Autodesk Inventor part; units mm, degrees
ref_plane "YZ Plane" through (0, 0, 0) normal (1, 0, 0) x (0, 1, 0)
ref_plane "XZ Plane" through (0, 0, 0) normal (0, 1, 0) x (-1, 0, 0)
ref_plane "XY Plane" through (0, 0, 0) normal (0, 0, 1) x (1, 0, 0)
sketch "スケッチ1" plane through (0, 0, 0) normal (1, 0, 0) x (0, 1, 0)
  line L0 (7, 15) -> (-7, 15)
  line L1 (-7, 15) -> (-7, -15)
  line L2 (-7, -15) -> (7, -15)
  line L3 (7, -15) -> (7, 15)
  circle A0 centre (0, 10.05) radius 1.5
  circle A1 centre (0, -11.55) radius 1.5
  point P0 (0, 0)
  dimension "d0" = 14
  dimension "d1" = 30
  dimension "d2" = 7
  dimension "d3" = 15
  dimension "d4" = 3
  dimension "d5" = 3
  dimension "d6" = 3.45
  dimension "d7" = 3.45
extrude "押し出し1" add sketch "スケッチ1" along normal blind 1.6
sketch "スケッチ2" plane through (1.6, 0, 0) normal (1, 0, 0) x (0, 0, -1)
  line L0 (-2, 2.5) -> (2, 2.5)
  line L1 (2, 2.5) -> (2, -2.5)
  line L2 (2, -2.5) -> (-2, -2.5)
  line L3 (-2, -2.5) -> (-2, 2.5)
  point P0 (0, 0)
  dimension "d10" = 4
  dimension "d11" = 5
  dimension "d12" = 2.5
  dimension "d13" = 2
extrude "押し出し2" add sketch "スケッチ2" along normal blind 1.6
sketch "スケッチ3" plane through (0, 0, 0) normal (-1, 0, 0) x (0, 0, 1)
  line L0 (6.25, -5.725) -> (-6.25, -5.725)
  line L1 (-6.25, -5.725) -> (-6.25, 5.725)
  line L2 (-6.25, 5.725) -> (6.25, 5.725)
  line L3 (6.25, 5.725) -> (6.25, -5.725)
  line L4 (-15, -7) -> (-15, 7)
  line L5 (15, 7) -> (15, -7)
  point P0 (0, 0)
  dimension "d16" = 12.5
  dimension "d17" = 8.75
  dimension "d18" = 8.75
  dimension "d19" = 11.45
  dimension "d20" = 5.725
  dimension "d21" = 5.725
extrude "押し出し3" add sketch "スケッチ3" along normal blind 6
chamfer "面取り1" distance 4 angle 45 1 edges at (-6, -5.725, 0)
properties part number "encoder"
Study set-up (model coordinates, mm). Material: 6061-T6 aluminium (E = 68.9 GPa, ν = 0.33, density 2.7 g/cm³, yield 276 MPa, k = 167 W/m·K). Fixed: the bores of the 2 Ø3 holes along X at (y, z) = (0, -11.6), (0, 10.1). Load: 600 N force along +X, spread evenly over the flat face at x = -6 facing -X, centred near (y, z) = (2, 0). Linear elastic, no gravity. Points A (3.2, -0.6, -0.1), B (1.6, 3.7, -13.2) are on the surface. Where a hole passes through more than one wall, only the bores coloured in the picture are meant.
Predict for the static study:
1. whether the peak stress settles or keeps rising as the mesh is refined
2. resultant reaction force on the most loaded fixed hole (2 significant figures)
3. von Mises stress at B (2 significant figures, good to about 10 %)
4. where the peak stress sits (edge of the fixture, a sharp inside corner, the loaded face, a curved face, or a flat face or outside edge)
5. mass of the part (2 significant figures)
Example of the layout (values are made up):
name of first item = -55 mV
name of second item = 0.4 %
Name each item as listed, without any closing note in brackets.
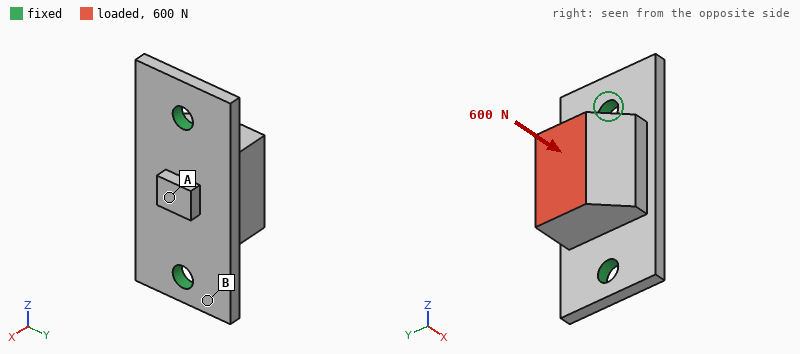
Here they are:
whether the peak stress settles or keeps rising as the mesh is refined = keeps rising
resultant reaction force on the most loaded fixed hole = 350 N
von Mises stress at B = 59 MPa
where the peak stress sits = edge of the fixture
mass of the part = 3.9 g
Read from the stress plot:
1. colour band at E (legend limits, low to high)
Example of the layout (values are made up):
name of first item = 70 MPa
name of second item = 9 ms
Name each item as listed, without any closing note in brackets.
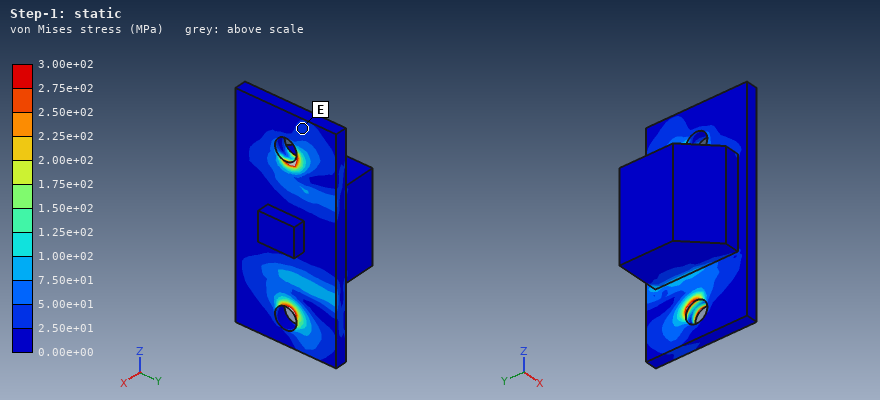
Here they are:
colour band at E = 2.50e+01 to 5.00e+01 MPa
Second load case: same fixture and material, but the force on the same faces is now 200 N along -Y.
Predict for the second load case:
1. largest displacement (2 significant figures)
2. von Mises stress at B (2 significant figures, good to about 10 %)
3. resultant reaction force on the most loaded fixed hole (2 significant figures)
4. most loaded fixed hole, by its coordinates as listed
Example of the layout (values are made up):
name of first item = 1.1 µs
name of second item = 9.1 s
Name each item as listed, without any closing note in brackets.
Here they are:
largest displacement = 38 µm
von Mises stress at B = 37 MPa
resultant reaction force on the most loaded fixed hole = 110 N
most loaded fixed hole, by its coordinates as listed = (0, 10.1)
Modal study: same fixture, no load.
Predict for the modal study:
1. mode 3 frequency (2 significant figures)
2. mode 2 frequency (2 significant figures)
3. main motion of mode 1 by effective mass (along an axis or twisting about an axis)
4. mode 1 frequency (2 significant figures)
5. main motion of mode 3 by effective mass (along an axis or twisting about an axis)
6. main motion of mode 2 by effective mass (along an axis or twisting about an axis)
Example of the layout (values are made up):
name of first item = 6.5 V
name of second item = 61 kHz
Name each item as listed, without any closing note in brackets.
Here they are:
mode 3 frequency = 30 kHz
mode 2 frequency = 17 kHz
main motion of mode 1 by effective mass = along Y
mode 1 frequency = 11 kHz
main motion of mode 3 by effective mass = along Z
main motion of mode 2 by effective mass = along X
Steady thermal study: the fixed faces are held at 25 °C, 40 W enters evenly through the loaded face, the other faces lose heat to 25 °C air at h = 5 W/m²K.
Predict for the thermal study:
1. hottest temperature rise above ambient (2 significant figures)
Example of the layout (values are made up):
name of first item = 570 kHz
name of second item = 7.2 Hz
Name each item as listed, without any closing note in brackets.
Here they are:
hottest temperature rise above ambient = 50 K
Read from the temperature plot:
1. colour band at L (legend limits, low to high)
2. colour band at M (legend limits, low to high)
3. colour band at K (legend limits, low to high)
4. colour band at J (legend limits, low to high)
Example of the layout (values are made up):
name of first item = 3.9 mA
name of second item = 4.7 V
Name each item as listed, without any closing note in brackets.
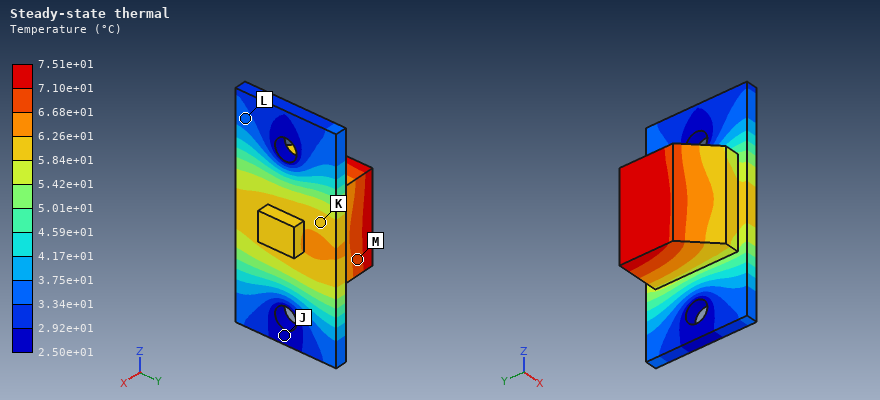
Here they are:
colour band at L = 3.34e+01 to 3.75e+01 °C
colour band at M = 6.68e+01 to 7.10e+01 °C
colour band at K = 5.84e+01 to 6.26e+01 °C
colour band at J = 2.50e+01 to 2.92e+01 °C
